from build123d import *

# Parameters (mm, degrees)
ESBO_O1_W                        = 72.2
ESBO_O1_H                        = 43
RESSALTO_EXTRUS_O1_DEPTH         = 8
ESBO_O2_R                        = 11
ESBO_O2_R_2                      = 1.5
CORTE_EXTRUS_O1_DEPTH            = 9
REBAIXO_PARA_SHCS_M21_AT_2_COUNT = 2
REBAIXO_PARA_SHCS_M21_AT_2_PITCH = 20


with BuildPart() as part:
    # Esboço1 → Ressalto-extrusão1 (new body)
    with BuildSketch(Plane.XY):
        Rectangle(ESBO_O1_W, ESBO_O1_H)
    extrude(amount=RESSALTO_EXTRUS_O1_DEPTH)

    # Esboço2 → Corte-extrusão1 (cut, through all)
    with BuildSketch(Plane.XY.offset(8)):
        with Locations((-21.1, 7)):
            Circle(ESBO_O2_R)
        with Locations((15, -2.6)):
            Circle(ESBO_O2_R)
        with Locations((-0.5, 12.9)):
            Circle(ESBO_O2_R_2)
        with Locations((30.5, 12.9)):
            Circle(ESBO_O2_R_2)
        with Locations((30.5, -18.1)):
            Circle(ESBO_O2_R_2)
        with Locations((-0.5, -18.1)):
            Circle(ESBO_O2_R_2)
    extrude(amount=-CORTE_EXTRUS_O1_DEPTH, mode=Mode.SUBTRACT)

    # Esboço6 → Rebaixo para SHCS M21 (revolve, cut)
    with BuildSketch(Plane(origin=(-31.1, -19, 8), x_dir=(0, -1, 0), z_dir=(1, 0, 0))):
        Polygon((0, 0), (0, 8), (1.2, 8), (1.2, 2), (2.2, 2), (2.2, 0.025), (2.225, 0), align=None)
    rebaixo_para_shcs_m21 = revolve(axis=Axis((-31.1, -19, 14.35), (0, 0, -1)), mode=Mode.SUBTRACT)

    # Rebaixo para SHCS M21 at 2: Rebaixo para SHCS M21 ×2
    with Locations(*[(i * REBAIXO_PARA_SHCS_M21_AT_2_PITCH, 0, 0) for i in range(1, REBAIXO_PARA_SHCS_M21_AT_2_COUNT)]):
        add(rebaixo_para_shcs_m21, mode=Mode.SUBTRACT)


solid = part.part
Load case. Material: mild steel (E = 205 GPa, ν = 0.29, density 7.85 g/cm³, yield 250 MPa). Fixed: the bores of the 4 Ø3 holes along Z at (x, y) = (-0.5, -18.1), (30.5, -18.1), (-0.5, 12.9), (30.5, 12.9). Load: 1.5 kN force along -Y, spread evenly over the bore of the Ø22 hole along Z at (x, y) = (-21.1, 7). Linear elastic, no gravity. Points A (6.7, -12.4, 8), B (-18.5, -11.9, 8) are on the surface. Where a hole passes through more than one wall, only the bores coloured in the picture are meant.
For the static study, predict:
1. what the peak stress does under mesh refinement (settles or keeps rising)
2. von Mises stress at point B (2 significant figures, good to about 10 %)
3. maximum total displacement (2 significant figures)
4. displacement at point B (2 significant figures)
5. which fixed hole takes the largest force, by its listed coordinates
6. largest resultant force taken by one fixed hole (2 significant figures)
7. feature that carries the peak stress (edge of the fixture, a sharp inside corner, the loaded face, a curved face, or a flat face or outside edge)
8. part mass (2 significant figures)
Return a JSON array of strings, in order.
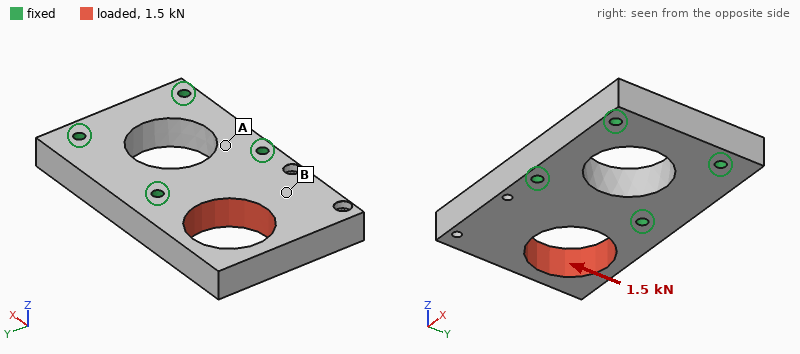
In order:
["keeps rising", "10 MPa", "8.3 µm", "2.6 µm", "(-0.5, 12.9)", "1.2 kN", "a sharp inside corner", "140 g"]
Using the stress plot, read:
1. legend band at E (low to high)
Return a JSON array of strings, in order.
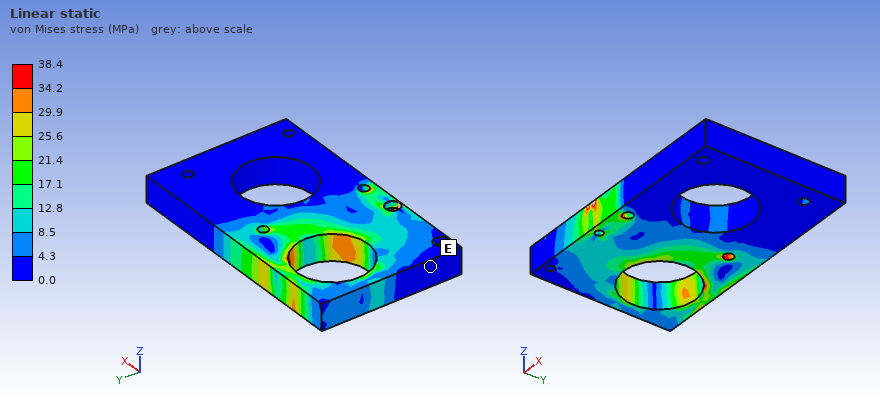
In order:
["0.0 to 4.3 MPa"]
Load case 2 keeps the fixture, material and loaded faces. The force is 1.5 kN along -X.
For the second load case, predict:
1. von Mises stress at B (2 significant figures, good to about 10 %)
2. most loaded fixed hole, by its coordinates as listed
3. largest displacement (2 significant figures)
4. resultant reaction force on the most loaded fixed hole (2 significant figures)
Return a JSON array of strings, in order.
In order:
["2.8 MPa", "(-0.5, 12.9)", "4.4 µm", "1.0 kN"]
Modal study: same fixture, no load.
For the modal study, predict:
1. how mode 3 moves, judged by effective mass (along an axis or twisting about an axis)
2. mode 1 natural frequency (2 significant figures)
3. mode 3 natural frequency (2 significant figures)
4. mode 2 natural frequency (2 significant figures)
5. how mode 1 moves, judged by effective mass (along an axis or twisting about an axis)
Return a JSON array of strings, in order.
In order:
["along Y", "4300 Hz", "11 kHz", "8200 Hz", "along Z"]
